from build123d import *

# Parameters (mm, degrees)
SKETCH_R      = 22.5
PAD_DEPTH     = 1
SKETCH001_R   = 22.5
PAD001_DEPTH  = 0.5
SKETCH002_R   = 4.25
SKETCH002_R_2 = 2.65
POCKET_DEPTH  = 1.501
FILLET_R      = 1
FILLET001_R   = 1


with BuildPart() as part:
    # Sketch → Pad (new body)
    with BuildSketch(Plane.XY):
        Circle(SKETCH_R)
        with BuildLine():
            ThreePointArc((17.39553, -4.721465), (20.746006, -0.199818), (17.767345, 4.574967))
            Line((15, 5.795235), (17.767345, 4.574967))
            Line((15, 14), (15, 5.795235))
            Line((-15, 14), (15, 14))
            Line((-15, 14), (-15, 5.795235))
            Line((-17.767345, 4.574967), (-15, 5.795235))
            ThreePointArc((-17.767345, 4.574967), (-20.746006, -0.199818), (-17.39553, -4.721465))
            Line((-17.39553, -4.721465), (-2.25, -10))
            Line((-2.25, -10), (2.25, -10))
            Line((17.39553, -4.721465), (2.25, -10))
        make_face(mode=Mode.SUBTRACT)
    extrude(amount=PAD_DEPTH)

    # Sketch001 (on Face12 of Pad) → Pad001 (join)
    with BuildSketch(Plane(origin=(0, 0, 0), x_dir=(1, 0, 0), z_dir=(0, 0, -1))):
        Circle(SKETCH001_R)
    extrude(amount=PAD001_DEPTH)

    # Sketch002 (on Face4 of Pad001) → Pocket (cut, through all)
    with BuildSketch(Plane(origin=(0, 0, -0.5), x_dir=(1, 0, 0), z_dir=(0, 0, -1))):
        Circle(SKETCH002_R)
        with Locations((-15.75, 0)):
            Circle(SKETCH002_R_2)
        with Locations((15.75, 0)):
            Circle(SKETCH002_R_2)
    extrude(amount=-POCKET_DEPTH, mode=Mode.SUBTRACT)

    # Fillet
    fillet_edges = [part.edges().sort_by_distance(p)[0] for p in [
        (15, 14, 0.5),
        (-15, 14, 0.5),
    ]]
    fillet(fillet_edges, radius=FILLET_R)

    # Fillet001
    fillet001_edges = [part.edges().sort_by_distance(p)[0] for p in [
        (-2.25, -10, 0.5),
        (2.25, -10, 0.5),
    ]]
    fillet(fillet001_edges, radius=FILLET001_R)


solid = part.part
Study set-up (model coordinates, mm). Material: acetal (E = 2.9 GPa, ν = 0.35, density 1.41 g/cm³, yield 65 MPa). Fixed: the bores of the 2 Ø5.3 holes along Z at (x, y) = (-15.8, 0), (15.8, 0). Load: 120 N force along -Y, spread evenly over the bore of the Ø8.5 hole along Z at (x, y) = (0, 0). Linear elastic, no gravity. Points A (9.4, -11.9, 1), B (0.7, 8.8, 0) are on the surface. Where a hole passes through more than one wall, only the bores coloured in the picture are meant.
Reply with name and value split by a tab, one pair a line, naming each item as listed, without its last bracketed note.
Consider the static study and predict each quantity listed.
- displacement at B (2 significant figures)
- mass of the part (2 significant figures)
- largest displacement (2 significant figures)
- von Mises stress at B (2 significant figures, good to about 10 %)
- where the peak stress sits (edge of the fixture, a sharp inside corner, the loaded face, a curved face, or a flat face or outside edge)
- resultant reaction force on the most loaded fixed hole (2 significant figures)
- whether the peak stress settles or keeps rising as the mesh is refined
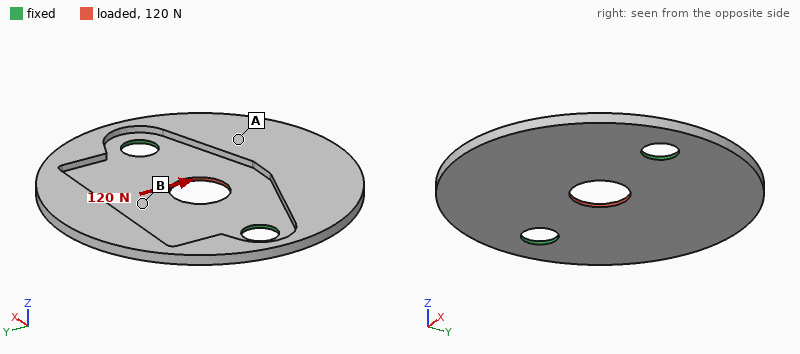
displacement at B	0.067 mm
mass of the part	2.2 g
largest displacement	0.13 mm
von Mises stress at B	7.9 MPa
where the peak stress sits	edge of the fixture
resultant reaction force on the most loaded fixed hole	60 N
whether the peak stress settles or keeps rising as the mesh is refined	keeps rising
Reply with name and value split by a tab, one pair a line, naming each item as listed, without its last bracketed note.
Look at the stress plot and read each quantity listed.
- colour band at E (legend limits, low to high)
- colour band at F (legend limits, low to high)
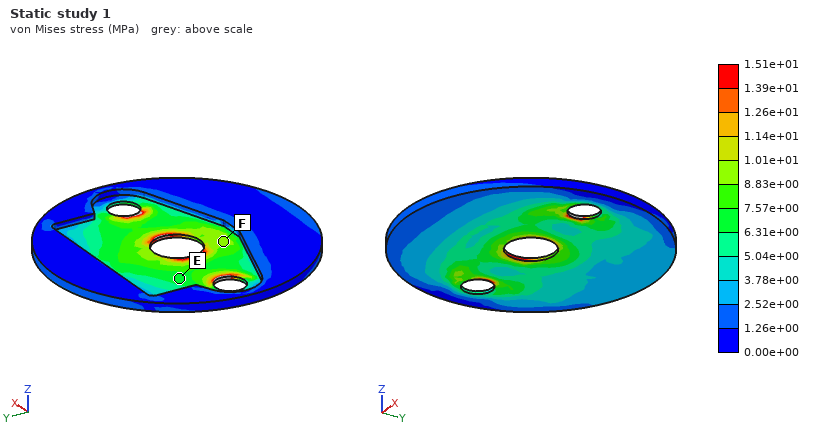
colour band at E	6.31e+00 to 7.57e+00 MPa
colour band at F	8.83e+00 to 1.01e+01 MPa
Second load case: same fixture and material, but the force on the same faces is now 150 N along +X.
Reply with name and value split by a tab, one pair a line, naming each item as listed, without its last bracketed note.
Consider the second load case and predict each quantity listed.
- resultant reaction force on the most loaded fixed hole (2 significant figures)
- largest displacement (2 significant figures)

resultant reaction force on the most loaded fixed hole	75 N
largest displacement	53 µm
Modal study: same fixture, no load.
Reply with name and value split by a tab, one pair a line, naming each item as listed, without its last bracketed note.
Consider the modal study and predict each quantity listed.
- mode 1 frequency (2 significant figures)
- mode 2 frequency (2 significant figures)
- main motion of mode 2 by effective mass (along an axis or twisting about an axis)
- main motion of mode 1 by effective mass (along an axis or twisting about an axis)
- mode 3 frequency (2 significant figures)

mode 1 frequency	370 Hz
mode 2 frequency	440 Hz
main motion of mode 2 by effective mass	along Z
main motion of mode 1 by effective mass	twisting about X
mode 3 frequency	1100 Hz
